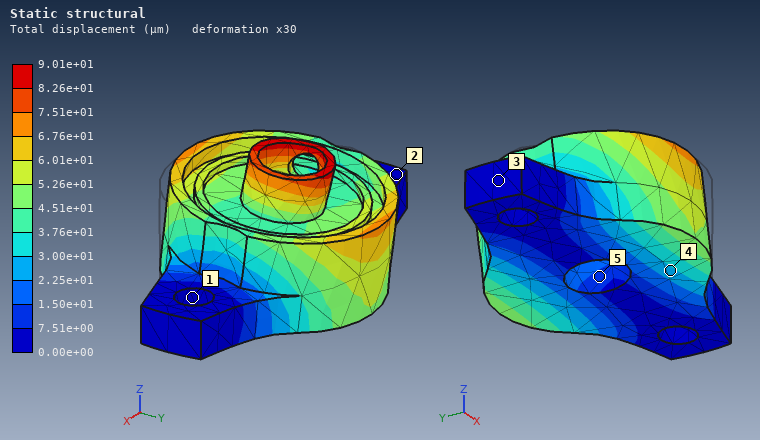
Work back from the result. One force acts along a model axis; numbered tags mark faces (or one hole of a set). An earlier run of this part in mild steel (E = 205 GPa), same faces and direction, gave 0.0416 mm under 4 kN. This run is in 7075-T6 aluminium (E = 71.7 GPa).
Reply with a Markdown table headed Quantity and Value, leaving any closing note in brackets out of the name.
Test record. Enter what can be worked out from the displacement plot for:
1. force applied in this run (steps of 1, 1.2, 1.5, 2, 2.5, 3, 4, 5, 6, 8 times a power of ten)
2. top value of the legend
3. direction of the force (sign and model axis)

| Quantity | Value |
|---|---|
| force applied in this run | 3 kN |
| top value of the legend | 9.01e+01 µm |
| direction of the force | +Y |
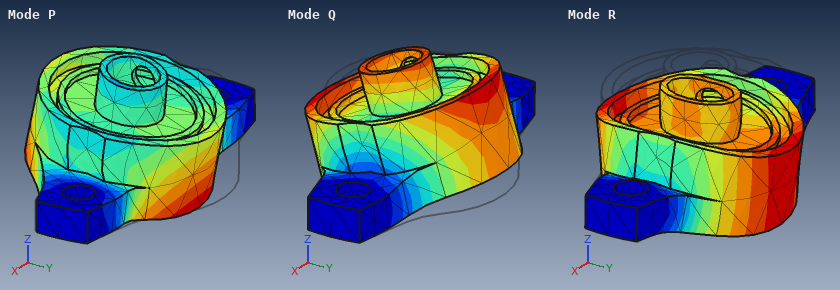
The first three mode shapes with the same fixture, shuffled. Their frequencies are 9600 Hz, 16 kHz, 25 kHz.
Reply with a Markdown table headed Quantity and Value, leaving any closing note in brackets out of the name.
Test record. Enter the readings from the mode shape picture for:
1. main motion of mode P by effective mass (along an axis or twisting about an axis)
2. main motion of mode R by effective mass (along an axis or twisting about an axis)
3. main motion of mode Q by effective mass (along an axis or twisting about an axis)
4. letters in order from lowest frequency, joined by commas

| Quantity | Value |
|---|---|
| main motion of mode P by effective mass | along Y |
| main motion of mode R by effective mass | along Z |
| main motion of mode Q by effective mass | along Y |
| letters in order from lowest frequency, joined by commas | Q, R, P |
